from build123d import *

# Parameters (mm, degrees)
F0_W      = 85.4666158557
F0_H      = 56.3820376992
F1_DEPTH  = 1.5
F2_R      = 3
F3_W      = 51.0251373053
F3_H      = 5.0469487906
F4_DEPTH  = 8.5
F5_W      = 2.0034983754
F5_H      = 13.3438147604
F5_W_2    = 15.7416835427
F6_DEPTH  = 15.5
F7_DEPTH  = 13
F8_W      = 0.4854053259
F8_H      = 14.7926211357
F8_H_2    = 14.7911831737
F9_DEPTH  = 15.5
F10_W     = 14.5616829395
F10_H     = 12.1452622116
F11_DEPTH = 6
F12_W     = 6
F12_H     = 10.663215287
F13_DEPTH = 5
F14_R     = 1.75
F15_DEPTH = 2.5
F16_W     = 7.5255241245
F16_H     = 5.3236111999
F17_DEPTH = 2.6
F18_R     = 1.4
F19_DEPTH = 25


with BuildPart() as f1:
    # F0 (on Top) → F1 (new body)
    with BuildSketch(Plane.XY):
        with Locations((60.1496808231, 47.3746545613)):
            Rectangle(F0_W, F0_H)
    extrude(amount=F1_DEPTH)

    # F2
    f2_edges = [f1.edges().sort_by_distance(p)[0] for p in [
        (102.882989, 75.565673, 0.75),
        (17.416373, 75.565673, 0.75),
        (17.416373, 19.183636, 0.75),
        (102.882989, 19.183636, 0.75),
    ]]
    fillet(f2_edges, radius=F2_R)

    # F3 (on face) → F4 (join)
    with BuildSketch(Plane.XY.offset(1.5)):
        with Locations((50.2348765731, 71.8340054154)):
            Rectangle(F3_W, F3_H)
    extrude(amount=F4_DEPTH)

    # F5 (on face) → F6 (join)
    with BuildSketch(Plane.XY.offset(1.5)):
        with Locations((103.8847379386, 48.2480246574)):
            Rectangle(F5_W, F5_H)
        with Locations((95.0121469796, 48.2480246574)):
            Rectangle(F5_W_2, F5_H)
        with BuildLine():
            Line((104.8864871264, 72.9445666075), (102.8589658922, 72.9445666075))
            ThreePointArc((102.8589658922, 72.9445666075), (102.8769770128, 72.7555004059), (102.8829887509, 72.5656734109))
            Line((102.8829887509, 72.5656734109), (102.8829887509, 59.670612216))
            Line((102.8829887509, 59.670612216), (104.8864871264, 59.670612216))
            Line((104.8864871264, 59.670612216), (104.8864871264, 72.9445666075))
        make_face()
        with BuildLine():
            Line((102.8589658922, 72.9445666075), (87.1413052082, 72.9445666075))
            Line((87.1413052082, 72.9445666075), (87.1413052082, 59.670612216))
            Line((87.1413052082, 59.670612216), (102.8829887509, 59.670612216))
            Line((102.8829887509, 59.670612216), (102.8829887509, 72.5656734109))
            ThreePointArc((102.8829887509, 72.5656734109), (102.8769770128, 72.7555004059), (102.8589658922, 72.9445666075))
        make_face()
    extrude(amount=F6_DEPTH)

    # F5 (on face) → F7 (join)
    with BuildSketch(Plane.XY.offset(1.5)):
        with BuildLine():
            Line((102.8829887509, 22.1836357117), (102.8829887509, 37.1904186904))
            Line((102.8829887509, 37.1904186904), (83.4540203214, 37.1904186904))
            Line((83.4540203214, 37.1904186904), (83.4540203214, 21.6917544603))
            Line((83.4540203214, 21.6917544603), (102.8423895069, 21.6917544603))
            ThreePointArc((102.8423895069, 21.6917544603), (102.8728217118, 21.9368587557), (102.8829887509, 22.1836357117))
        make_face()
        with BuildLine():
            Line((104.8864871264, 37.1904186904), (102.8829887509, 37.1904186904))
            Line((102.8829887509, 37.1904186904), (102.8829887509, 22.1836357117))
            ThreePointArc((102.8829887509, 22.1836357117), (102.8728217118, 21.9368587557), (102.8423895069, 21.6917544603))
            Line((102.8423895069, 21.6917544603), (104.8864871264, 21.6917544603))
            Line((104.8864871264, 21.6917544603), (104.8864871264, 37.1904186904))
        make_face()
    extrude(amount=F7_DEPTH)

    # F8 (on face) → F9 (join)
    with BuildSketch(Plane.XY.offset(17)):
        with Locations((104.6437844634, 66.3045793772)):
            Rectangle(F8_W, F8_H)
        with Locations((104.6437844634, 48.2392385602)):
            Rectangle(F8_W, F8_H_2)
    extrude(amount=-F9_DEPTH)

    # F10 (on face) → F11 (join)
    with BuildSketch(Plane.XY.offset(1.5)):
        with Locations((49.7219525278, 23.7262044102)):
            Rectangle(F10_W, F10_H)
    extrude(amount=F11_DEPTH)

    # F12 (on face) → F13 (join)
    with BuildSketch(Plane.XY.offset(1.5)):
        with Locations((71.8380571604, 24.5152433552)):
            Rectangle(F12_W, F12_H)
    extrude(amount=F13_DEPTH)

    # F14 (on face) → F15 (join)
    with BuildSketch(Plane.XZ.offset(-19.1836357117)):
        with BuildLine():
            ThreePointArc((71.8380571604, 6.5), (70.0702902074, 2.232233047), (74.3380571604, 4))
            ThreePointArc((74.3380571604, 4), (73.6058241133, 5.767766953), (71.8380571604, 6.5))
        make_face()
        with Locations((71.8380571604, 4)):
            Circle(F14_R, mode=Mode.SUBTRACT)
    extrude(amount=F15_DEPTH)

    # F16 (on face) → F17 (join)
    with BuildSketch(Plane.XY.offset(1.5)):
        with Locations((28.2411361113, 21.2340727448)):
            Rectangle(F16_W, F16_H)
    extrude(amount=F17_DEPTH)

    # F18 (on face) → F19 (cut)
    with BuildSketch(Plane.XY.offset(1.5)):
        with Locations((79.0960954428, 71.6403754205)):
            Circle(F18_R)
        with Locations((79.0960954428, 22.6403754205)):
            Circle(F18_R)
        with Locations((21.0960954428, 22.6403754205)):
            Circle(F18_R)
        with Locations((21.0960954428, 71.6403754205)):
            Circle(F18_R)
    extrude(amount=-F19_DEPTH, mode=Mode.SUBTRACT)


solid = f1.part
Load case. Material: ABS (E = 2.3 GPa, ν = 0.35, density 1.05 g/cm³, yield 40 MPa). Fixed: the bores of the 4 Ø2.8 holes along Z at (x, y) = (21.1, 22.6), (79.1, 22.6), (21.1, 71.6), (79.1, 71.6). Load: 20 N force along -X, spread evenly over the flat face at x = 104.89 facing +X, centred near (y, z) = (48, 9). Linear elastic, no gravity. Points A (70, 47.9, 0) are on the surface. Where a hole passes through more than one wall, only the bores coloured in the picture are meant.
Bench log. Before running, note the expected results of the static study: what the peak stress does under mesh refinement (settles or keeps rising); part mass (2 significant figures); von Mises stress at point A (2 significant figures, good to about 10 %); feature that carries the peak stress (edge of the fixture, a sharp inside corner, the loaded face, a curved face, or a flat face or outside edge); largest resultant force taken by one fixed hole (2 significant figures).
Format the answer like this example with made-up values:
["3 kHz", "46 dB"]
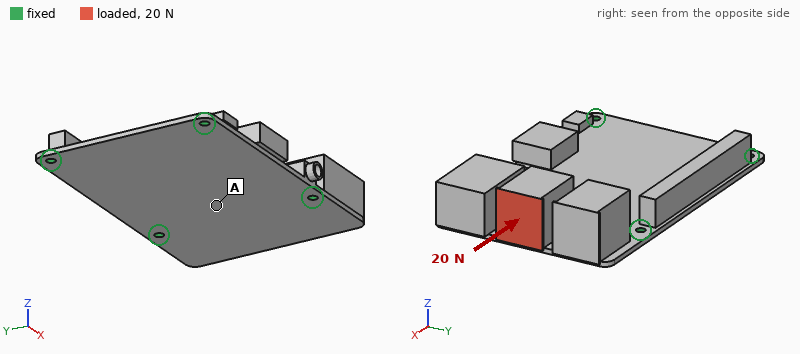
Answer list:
["keeps rising", "24 g", "1.8 MPa", "edge of the fixture", "7.4 N"]
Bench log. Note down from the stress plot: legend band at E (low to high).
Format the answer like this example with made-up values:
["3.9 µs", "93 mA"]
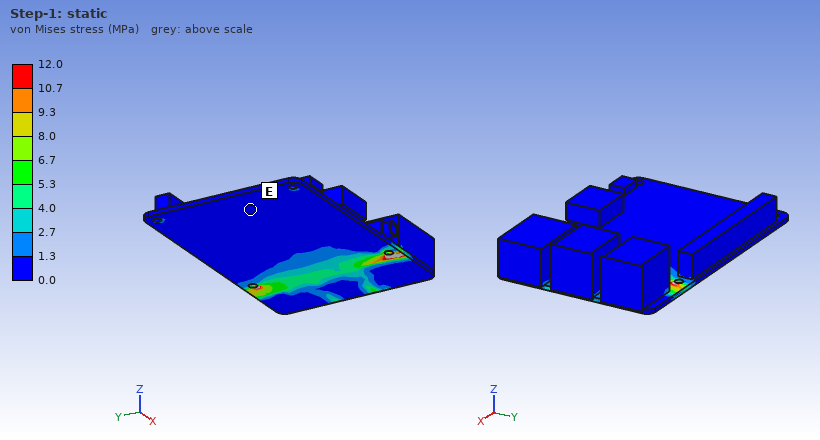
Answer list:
["0.0 to 1.3 MPa"]
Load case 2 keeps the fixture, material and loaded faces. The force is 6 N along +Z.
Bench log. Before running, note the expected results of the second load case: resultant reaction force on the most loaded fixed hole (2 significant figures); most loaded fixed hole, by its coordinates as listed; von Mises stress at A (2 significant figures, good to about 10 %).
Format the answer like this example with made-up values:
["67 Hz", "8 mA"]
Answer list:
["3.9 N", "(79.1, 71.6)", "1.8 MPa"]
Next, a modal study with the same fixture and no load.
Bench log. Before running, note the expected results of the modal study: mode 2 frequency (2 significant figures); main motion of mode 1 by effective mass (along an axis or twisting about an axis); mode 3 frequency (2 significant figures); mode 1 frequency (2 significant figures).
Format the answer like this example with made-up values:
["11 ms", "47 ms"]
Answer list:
["500 Hz", "along Z", "570 Hz", "160 Hz"]
